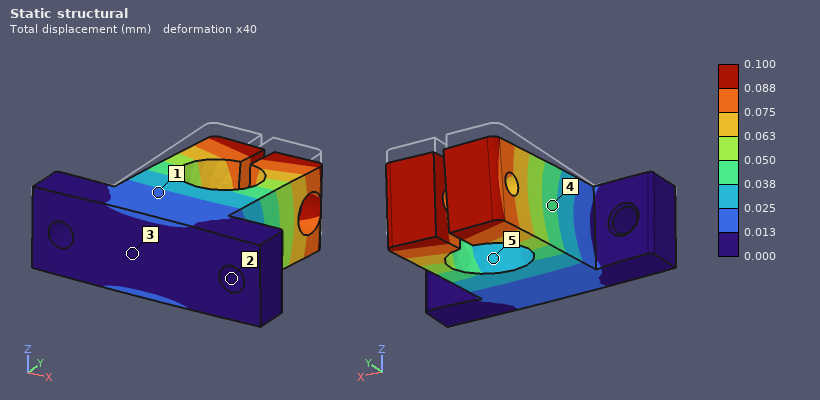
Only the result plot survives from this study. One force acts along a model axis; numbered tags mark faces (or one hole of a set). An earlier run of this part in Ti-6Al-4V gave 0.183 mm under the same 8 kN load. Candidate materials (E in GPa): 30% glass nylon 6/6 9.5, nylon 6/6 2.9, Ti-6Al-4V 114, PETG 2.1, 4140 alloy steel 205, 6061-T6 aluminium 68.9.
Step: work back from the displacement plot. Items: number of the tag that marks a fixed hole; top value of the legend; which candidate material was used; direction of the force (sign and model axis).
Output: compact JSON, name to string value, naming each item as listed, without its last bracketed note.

{"number of the tag that marks a fixed hole": "2", "top value of the legend": "0.100 mm", "which candidate material was used": "4140 alloy steel", "direction of the force": "-Z"}
